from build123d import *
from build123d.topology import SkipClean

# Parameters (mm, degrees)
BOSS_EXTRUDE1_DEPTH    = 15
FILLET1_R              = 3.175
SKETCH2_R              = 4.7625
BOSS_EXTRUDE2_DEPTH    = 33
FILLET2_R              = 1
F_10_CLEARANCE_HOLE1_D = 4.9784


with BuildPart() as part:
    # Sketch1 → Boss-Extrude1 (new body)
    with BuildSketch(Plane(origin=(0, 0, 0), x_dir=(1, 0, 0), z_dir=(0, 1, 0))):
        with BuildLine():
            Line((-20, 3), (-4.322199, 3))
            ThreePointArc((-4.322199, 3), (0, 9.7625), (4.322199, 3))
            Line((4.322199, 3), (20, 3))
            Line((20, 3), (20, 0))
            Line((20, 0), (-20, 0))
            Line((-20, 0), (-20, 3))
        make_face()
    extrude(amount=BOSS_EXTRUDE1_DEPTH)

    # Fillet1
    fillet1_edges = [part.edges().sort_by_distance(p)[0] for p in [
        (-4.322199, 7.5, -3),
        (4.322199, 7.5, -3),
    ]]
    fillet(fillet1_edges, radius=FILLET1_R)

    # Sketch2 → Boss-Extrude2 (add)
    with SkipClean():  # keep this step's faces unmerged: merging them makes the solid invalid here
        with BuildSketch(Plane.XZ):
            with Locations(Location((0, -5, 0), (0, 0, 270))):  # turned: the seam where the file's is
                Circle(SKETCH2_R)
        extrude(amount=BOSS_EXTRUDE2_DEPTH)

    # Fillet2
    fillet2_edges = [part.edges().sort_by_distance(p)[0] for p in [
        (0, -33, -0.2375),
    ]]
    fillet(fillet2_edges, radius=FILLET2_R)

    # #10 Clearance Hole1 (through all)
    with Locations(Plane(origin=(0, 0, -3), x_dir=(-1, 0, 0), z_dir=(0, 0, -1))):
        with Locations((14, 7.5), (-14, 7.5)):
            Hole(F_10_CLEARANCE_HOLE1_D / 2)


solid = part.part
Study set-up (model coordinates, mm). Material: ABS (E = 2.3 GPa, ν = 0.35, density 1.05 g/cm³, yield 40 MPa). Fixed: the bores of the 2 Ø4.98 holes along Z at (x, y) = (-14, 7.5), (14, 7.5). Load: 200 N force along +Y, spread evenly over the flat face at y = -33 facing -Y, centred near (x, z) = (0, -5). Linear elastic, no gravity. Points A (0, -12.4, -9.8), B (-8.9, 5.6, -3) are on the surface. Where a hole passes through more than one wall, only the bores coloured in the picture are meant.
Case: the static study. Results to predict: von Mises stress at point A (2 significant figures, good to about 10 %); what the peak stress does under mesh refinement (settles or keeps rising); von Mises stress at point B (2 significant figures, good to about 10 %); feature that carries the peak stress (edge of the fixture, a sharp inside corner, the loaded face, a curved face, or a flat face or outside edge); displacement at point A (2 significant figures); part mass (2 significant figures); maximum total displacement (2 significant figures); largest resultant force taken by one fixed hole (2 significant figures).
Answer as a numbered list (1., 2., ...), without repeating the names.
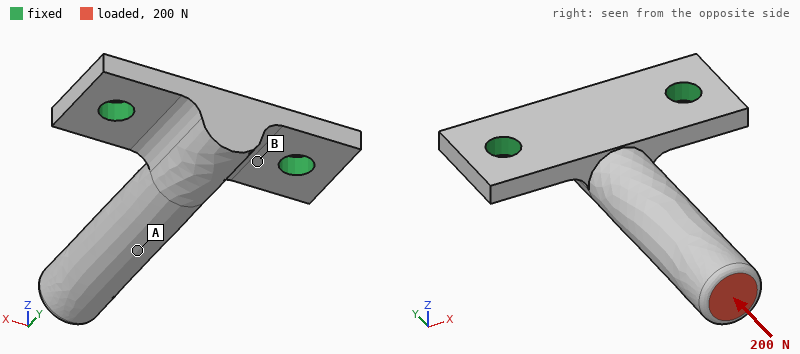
1. 2.8 MPa
2. keeps rising
3. 14 MPa
4. edge of the fixture
5. 0.41 mm
6. 5.2 g
7. 0.76 mm
8. 100 N
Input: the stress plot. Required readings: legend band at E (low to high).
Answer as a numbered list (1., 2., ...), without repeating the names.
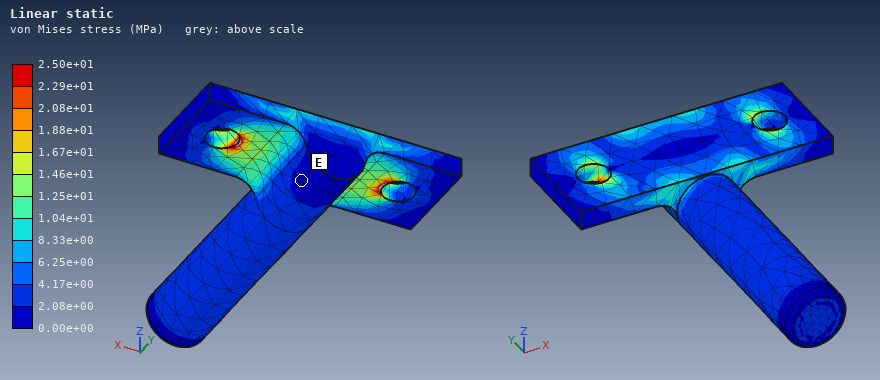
1. 0.00e+00 to 2.08e+00 MPa
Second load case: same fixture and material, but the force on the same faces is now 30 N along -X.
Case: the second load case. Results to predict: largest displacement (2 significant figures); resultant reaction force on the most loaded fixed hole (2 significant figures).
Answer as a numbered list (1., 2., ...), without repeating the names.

1. 0.60 mm
2. 49 N
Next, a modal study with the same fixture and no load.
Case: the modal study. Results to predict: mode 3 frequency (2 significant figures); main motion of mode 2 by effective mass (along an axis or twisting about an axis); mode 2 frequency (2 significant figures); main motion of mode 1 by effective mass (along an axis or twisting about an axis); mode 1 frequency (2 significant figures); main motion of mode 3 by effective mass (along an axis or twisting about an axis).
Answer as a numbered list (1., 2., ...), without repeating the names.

1. 4200 Hz
2. along X
3. 1400 Hz
4. along Z
5. 690 Hz
6. along Y
